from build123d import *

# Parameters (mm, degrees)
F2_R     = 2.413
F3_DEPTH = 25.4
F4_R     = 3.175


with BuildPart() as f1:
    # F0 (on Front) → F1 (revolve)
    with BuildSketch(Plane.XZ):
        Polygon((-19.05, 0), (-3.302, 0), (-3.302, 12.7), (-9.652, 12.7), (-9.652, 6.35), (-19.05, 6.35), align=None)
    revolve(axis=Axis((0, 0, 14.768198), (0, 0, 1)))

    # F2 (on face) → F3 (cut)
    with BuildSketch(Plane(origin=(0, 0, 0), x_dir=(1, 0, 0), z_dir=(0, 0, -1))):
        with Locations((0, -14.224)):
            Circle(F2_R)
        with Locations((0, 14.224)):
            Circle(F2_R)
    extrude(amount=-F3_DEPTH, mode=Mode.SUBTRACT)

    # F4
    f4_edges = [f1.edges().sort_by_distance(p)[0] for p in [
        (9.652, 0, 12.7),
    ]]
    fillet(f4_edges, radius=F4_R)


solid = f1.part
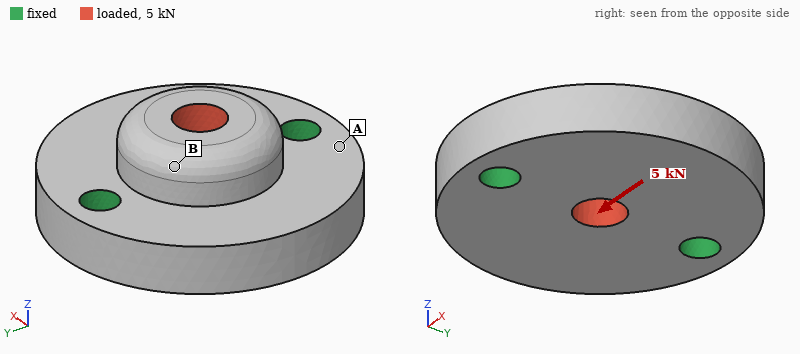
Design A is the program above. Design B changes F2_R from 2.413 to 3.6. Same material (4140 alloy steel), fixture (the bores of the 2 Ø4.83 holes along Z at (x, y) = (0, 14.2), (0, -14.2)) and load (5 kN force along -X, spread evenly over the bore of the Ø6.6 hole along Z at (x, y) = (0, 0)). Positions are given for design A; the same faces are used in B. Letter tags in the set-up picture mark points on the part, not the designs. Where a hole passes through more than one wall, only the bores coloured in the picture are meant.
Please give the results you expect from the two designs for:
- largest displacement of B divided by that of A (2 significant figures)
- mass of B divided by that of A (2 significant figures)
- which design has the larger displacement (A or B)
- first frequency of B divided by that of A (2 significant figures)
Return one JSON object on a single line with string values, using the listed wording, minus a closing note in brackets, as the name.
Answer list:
{"largest displacement of B divided by that of A": "0.67", "mass of B divided by that of A": "0.97", "which design has the larger displacement": "A", "first frequency of B divided by that of A": "1.2"}
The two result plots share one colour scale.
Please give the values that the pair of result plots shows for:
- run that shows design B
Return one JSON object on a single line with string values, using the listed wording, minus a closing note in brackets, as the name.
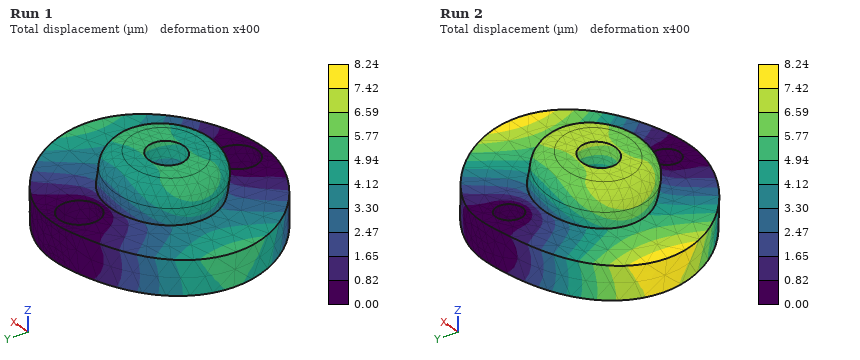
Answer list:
{"run that shows design B": "Run 1"}
